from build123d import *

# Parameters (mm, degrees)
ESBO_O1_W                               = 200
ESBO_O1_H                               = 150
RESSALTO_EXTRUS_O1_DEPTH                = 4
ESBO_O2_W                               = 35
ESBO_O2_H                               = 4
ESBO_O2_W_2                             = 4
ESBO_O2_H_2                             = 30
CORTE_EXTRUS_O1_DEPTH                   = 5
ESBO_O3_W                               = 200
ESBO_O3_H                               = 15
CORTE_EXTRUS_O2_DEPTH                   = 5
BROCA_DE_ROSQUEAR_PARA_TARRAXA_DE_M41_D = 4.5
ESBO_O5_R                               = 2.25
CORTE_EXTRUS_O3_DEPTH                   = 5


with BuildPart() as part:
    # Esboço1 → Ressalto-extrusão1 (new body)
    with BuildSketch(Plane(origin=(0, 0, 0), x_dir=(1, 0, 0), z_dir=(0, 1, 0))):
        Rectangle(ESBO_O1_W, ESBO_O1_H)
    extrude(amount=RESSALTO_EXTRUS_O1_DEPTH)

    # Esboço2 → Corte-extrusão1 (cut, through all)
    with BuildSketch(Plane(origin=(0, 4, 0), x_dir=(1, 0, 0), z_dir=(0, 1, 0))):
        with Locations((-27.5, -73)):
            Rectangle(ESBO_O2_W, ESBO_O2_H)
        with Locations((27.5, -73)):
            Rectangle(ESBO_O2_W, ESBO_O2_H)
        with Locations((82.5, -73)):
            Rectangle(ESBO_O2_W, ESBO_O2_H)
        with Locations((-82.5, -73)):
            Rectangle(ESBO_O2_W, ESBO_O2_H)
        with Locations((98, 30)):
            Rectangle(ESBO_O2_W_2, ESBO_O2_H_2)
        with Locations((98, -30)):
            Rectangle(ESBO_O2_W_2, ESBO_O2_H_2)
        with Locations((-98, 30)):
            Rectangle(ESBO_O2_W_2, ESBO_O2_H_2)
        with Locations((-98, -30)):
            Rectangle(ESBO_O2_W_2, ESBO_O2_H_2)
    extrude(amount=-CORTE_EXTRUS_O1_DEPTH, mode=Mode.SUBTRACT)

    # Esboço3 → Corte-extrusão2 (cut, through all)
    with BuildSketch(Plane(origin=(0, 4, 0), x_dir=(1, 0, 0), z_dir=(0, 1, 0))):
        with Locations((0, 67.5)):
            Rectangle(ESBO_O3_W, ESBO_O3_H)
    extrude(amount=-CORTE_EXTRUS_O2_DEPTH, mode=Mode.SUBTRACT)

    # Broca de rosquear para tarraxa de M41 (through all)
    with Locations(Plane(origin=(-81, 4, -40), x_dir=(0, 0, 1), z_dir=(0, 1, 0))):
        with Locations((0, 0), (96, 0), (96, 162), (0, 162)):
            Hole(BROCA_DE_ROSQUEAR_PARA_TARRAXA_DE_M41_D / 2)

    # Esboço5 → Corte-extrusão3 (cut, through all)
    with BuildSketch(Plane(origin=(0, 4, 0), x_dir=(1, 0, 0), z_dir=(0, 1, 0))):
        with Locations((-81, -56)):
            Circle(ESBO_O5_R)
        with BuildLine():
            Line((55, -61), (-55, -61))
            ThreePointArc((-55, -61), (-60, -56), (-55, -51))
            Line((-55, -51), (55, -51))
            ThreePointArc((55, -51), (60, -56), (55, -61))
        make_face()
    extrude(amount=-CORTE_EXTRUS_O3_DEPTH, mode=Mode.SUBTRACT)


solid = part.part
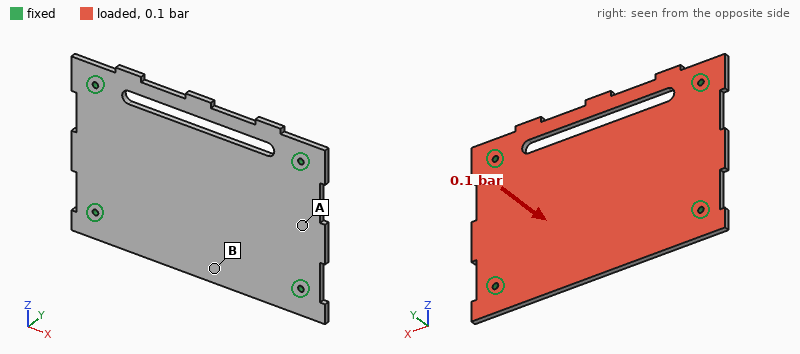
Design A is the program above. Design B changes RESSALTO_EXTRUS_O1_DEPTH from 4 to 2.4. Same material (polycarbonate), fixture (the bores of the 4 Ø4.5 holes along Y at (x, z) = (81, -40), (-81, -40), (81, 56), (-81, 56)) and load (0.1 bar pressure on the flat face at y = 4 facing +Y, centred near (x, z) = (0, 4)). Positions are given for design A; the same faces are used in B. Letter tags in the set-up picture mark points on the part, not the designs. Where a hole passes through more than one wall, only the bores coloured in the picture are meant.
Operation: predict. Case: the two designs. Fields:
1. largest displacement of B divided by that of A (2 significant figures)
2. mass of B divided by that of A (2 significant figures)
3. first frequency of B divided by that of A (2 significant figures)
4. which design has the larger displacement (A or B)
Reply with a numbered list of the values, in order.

1. 4.4
2. 0.60
3. 0.62
4. B
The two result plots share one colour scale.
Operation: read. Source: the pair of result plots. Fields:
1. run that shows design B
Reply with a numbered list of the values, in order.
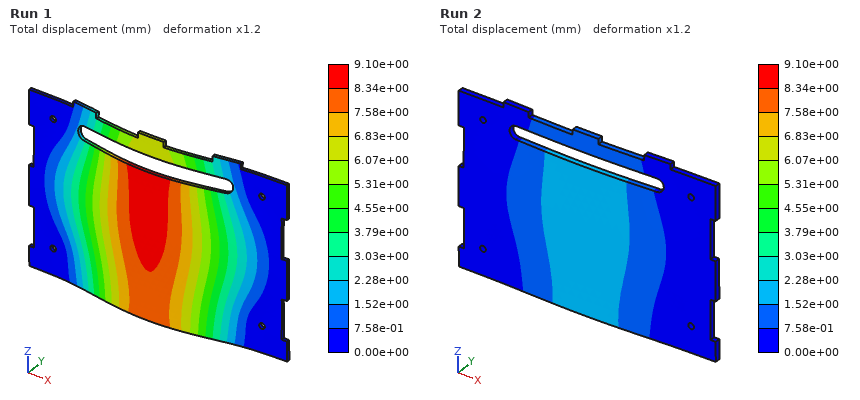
1. Run 1
